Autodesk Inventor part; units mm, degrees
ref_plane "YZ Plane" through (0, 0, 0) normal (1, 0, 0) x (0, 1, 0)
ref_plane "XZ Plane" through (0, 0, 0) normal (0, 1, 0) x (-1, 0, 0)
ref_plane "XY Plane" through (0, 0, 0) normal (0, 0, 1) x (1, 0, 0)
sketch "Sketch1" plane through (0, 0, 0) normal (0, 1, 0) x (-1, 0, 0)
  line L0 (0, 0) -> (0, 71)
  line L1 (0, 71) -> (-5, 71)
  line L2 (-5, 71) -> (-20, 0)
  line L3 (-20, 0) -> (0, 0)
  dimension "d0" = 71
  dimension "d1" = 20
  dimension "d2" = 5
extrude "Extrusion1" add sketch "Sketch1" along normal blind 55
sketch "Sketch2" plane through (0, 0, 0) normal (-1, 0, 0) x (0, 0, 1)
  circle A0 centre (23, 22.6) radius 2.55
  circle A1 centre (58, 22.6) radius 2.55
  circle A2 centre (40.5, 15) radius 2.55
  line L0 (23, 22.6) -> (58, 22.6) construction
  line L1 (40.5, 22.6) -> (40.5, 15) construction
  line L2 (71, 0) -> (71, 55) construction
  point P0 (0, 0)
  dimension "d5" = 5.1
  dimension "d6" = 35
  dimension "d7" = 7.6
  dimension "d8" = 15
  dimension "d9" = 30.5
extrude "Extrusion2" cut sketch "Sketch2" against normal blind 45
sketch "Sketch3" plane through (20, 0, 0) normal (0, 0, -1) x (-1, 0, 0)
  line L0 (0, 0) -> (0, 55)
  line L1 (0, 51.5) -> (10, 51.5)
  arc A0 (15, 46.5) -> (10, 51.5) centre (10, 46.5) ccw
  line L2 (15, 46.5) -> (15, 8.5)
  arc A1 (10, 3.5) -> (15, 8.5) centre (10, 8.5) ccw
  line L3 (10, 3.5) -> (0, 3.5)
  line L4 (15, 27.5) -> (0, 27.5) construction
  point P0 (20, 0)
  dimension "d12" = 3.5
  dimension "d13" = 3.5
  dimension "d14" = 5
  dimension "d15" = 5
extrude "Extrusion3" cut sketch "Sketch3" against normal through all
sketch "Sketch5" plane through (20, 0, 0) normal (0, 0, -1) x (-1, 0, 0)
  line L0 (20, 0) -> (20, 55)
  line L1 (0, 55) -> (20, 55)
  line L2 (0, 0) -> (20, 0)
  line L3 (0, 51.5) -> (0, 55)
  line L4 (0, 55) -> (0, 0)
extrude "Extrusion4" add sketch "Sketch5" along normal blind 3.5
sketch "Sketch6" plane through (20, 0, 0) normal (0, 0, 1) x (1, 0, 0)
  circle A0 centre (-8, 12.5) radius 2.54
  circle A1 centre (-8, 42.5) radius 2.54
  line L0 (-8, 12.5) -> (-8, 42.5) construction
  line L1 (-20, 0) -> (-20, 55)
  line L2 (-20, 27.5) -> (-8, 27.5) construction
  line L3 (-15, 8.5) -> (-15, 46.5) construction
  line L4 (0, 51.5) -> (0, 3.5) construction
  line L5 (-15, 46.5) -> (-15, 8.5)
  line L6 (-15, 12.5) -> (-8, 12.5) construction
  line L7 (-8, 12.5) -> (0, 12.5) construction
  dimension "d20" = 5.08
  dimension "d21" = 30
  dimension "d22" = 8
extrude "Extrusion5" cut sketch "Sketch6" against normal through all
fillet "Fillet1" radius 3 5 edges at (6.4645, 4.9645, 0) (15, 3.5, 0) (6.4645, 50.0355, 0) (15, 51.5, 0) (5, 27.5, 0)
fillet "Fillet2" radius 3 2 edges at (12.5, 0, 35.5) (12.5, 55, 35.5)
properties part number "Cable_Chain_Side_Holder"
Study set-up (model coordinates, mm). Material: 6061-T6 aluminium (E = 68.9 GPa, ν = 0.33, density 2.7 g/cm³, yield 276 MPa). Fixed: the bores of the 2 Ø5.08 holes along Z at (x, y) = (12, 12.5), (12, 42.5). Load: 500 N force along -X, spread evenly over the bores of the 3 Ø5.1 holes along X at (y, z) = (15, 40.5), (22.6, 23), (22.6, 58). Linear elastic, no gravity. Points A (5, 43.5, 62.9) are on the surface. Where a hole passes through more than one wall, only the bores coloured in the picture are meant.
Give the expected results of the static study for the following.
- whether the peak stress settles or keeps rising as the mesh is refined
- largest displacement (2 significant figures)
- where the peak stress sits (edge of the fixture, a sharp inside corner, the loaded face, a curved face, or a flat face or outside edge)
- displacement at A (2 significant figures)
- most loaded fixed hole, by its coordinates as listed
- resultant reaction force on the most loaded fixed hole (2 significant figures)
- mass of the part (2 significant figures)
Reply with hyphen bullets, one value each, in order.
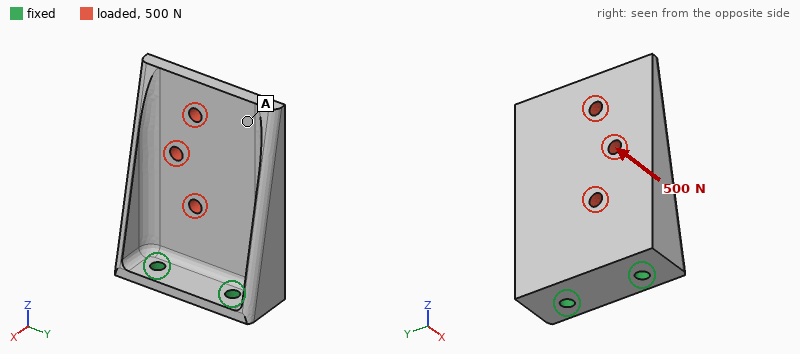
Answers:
- keeps rising
- 0.56 mm
- edge of the fixture
- 0.44 mm
- (12, 12.5)
- 360 N
- 73 g
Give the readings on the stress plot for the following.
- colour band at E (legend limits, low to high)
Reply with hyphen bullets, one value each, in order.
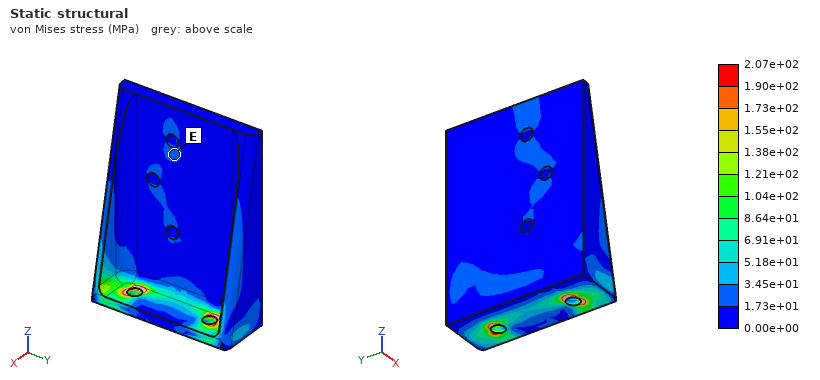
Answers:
- 1.73e+01 to 3.45e+01 MPa
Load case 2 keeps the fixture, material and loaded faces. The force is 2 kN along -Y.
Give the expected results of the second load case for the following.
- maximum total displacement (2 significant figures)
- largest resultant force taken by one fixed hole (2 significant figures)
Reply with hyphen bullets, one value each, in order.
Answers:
- 0.28 mm
- 2.7 kN
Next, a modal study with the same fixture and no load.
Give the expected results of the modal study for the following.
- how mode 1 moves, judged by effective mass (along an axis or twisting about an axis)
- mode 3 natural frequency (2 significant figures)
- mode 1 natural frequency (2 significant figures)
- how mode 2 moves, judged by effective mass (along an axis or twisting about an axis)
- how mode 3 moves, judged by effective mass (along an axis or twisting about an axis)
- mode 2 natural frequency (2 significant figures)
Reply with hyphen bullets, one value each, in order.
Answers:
- along X
- 3400 Hz
- 850 Hz
- along Y
- along Y
- 1900 Hz
